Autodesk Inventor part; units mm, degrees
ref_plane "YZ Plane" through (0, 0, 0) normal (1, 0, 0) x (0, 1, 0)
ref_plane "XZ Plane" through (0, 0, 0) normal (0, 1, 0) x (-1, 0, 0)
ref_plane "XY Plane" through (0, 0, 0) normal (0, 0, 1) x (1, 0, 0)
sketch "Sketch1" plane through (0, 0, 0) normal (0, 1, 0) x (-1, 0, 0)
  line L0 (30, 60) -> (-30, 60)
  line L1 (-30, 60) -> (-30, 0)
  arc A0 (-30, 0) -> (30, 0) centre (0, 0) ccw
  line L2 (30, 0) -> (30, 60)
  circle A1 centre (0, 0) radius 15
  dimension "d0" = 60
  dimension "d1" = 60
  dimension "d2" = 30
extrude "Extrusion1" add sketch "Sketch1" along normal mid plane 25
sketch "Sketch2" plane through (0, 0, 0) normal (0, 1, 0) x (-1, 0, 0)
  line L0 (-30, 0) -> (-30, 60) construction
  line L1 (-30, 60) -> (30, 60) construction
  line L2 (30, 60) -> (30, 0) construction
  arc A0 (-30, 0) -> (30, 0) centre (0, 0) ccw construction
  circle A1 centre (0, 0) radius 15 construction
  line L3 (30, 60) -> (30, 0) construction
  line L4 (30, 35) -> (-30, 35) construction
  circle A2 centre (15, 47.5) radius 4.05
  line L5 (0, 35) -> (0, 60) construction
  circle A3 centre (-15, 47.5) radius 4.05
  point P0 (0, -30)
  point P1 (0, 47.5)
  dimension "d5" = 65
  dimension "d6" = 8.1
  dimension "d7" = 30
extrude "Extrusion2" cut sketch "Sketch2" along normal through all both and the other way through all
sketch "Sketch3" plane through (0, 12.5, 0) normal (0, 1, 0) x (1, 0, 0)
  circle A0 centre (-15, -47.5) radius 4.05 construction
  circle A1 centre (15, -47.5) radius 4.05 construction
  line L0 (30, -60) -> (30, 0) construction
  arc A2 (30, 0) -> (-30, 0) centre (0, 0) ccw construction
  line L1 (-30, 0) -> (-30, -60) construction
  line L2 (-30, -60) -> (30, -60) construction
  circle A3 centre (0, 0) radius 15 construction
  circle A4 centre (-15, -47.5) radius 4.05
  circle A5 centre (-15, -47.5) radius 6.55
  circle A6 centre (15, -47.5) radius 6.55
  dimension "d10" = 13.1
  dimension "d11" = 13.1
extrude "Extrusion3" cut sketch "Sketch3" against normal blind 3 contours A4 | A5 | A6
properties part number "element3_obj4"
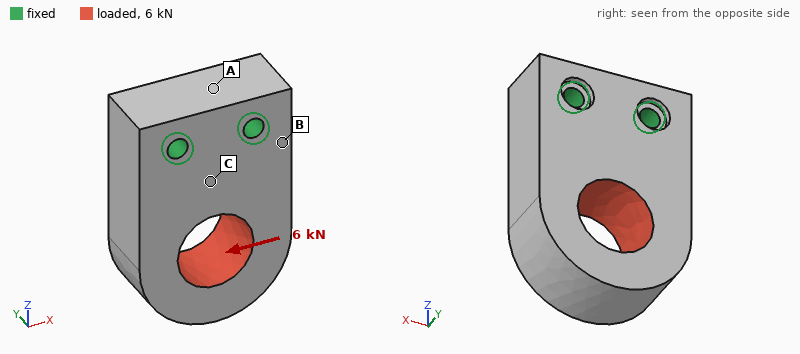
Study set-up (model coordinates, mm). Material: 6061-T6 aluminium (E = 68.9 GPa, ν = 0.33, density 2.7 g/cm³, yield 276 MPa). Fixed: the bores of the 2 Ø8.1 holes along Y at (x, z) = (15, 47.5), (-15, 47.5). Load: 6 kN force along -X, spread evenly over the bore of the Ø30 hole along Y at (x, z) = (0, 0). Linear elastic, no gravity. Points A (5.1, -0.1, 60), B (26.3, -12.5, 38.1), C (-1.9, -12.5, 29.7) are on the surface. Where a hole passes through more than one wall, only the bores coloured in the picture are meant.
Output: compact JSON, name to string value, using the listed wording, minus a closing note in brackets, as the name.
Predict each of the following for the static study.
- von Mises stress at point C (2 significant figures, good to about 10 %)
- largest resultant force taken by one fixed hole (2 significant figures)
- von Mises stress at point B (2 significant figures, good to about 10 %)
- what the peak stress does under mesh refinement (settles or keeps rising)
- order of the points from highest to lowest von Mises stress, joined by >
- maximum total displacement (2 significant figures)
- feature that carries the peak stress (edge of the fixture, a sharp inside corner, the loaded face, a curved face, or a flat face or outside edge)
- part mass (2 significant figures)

{"von Mises stress at point C": "19 MPa", "largest resultant force taken by one fixed hole": "8.3 kN", "von Mises stress at point B": "10 MPa", "what the peak stress does under mesh refinement": "keeps rising", "order of the points from highest to lowest von Mises stress, joined by >": "C > B > A", "maximum total displacement": "42 µm", "feature that carries the peak stress": "edge of the fixture", "part mass": "280 g"}
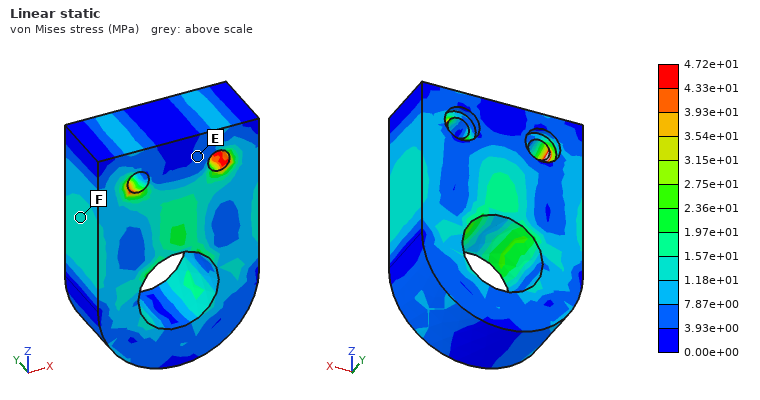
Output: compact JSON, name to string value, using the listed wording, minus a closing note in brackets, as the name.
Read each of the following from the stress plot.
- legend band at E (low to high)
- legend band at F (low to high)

{"legend band at E": "3.93e+00 to 7.87e+00 MPa", "legend band at F": "1.18e+01 to 1.57e+01 MPa"}
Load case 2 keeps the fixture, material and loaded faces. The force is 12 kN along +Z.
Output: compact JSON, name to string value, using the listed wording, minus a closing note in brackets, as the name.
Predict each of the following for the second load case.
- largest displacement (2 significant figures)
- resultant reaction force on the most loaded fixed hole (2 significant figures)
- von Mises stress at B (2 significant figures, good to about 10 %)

{"largest displacement": "15 µm", "resultant reaction force on the most loaded fixed hole": "6.0 kN", "von Mises stress at B": "6.3 MPa"}
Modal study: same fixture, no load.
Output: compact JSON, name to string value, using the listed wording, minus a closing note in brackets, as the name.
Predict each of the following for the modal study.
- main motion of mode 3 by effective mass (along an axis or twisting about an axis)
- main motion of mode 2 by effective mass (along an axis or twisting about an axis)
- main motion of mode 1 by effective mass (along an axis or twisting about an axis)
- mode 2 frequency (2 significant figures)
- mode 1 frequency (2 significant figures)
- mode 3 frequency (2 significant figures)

{"main motion of mode 3 by effective mass": "twisting about Z", "main motion of mode 2 by effective mass": "along X", "main motion of mode 1 by effective mass": "along Y", "mode 2 frequency": "5600 Hz", "mode 1 frequency": "3500 Hz", "mode 3 frequency": "7700 Hz"}
